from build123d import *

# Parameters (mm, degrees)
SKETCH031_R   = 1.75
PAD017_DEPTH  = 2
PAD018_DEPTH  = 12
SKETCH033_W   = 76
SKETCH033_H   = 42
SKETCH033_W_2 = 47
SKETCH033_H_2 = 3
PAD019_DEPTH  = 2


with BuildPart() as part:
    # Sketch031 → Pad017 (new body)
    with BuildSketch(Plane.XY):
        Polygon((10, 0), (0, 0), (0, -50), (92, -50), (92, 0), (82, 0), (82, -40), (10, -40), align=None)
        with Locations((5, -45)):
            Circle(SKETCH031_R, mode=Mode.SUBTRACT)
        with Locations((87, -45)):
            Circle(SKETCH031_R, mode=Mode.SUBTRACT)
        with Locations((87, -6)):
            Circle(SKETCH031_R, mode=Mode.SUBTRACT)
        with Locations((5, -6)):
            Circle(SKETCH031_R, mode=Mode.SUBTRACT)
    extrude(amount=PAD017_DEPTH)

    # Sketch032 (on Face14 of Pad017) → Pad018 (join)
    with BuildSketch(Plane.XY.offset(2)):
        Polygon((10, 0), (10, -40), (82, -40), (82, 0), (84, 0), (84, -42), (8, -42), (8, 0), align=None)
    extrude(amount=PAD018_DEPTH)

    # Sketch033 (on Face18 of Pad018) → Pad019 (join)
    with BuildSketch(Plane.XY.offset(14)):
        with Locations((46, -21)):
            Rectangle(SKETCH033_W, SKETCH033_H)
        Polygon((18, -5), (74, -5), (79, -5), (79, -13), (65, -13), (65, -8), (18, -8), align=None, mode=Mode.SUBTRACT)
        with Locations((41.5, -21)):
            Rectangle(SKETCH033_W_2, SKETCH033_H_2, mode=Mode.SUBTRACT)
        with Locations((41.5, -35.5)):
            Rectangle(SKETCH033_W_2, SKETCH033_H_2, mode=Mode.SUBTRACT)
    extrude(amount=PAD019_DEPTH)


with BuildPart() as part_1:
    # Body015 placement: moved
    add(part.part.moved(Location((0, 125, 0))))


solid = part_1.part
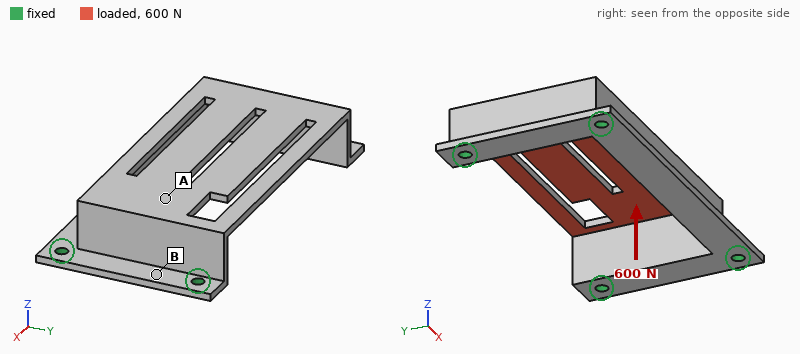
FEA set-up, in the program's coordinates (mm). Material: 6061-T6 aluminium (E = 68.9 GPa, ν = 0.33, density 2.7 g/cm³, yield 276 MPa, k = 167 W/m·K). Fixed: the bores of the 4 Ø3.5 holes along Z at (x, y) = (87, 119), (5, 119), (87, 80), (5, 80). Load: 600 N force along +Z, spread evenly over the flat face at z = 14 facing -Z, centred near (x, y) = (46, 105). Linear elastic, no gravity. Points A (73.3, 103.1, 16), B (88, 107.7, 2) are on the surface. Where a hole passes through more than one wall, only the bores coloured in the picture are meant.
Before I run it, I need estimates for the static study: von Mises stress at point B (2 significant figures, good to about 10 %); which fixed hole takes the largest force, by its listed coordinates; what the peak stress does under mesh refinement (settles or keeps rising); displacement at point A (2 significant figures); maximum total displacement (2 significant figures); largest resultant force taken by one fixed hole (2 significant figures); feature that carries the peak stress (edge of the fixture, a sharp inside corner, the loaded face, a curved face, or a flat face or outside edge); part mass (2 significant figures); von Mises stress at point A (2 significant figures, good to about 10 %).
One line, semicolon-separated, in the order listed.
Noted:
11 MPa; (5, 119); keeps rising; 0.082 mm; 0.47 mm; 280 N; a sharp inside corner; 34 g; 61 MPa
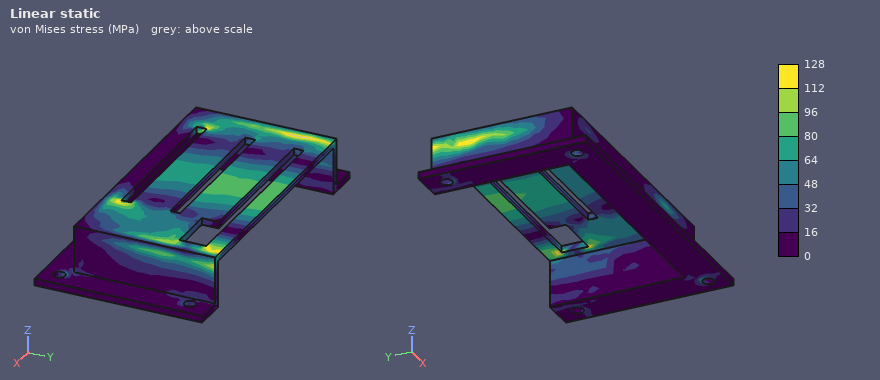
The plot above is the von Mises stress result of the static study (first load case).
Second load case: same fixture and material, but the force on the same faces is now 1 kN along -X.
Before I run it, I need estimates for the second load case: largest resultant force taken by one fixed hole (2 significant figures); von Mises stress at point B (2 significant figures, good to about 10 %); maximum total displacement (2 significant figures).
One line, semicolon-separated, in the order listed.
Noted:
520 N; 11 MPa; 77 µm
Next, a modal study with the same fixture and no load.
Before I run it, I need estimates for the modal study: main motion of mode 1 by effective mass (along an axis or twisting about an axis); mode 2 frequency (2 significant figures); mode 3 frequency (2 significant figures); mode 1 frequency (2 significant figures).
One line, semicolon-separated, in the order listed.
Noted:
along Z; 2200 Hz; 3100 Hz; 1900 Hz
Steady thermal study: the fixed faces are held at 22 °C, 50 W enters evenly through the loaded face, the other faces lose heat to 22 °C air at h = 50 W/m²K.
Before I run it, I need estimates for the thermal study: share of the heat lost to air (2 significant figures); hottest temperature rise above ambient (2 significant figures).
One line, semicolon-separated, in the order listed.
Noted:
27 %; 61 K
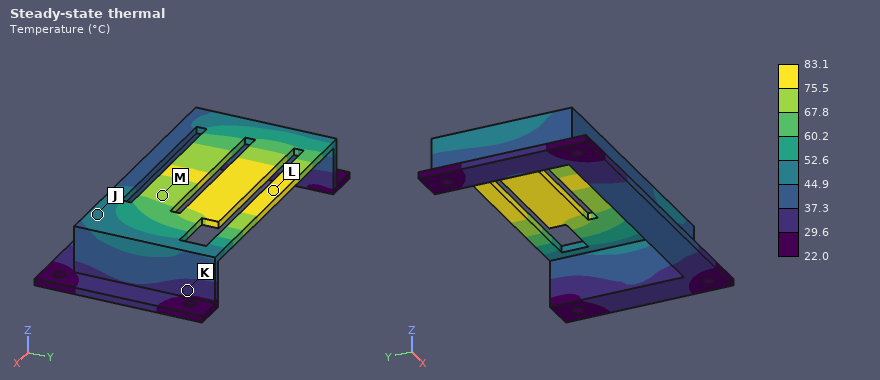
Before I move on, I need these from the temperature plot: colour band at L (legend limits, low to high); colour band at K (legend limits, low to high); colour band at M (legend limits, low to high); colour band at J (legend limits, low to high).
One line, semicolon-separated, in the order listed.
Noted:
75.5 to 83.1 °C; 29.6 to 37.3 °C; 67.8 to 75.5 °C; 44.9 to 52.6 °C
